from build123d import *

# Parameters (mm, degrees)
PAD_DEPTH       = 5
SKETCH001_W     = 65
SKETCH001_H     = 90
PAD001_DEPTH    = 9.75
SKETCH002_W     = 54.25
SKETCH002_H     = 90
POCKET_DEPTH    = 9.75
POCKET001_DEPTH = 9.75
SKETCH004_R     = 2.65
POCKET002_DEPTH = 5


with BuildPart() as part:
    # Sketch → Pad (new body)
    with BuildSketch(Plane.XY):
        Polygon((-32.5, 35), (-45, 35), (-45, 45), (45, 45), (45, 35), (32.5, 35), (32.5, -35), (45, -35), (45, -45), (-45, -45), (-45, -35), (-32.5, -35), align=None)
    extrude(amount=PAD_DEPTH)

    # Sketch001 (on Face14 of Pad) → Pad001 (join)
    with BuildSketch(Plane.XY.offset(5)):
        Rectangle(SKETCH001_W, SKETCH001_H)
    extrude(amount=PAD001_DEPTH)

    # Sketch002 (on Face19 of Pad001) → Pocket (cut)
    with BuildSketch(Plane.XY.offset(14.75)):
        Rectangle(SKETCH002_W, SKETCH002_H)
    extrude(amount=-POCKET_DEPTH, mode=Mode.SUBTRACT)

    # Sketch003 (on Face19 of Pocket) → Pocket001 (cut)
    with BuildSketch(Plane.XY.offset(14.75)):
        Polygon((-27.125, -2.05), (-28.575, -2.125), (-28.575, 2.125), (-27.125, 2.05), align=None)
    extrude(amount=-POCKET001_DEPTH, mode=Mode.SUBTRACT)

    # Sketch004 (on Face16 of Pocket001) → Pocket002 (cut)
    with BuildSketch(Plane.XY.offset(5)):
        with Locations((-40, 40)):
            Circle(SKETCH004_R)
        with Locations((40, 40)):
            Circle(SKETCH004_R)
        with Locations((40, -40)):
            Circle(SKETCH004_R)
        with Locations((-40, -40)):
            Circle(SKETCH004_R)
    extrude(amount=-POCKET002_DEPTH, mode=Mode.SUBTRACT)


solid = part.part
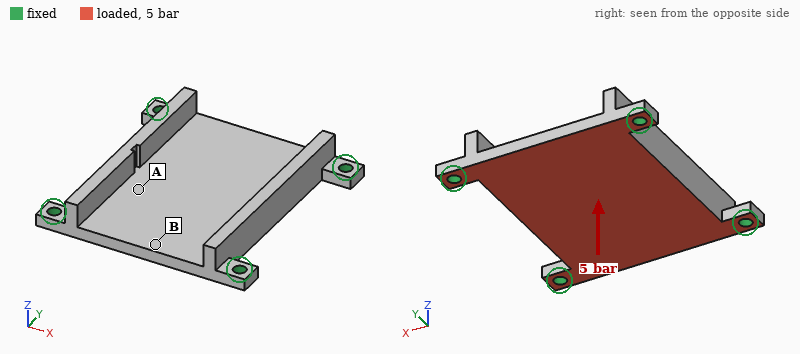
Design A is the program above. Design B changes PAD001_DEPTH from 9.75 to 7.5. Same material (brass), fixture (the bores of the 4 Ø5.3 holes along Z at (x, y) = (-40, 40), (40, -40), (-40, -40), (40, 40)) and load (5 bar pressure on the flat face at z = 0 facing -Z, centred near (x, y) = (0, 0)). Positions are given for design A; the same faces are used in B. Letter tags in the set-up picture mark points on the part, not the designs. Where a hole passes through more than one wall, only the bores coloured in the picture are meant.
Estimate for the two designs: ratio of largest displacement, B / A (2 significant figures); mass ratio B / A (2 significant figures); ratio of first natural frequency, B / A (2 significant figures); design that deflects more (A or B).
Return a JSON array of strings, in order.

["1.1", "0.95", "0.98", "B"]
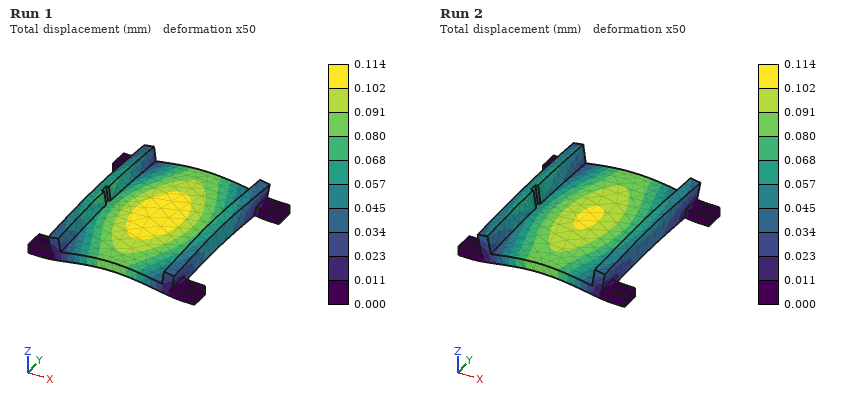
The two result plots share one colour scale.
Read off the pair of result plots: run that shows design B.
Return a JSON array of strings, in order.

["Run 1"]
